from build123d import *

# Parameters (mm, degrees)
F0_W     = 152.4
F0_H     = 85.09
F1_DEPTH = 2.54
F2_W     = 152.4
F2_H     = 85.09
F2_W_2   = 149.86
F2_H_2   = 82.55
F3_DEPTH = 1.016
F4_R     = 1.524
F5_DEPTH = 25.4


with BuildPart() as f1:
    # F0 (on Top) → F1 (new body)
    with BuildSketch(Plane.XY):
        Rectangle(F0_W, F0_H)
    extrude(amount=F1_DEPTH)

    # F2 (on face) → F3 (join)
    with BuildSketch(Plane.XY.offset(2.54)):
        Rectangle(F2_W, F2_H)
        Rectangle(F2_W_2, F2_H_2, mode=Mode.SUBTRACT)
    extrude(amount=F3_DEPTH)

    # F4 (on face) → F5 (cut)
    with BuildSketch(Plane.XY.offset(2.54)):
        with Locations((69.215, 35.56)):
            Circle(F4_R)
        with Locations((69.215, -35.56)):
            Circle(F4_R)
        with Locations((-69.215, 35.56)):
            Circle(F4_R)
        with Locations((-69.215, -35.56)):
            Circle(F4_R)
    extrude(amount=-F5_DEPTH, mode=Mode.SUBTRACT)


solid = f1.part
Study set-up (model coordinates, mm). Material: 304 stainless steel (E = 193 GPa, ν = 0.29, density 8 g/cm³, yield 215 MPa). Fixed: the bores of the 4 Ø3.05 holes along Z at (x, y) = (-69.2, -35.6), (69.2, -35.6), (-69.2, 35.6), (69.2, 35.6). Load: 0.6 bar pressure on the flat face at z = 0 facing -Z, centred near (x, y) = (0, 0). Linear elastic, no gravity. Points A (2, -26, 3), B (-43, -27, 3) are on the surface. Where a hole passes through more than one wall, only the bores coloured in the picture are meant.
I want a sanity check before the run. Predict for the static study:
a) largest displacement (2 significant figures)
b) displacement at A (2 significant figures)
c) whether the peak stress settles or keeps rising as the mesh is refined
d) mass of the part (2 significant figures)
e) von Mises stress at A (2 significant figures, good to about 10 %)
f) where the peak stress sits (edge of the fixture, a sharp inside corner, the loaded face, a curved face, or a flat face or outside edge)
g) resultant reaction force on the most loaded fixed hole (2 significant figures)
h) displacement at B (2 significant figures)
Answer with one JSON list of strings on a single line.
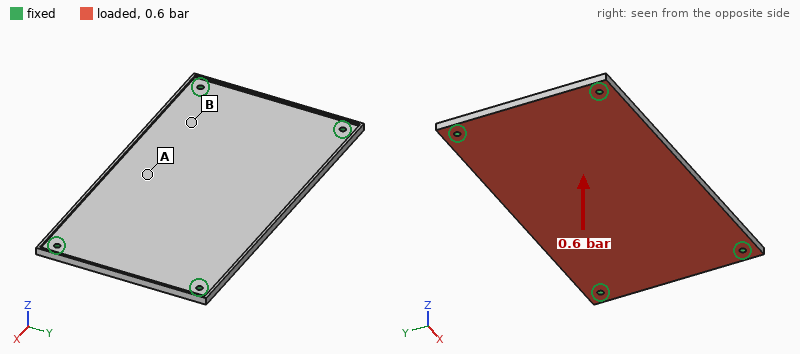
["0.29 mm", "0.28 mm", "keeps rising", "270 g", "46 MPa", "edge of the fixture", "190 N", "0.13 mm"]
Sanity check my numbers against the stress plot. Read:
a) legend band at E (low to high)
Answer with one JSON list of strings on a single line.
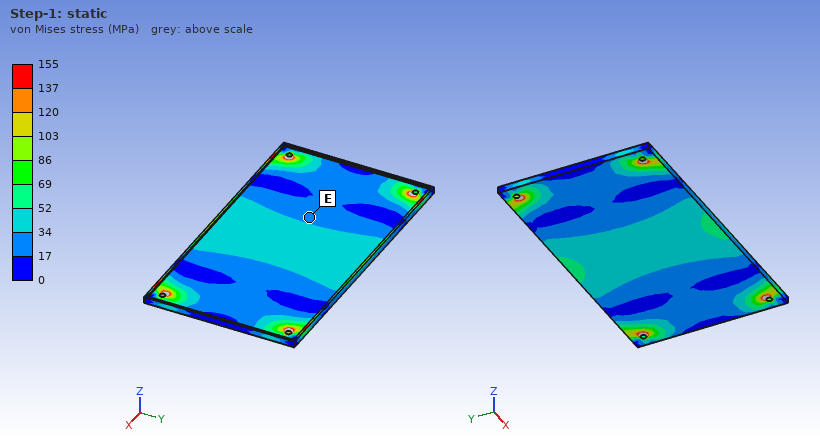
["17 to 34 MPa"]
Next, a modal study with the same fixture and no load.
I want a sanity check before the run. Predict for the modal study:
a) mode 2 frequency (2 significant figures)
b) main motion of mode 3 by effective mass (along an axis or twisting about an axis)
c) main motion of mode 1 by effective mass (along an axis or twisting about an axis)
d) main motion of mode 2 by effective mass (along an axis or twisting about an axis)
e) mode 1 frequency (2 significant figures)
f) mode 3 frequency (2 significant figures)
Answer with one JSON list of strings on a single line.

["990 Hz", "twisting about Y", "along Z", "twisting about X", "580 Hz", "1600 Hz"]
